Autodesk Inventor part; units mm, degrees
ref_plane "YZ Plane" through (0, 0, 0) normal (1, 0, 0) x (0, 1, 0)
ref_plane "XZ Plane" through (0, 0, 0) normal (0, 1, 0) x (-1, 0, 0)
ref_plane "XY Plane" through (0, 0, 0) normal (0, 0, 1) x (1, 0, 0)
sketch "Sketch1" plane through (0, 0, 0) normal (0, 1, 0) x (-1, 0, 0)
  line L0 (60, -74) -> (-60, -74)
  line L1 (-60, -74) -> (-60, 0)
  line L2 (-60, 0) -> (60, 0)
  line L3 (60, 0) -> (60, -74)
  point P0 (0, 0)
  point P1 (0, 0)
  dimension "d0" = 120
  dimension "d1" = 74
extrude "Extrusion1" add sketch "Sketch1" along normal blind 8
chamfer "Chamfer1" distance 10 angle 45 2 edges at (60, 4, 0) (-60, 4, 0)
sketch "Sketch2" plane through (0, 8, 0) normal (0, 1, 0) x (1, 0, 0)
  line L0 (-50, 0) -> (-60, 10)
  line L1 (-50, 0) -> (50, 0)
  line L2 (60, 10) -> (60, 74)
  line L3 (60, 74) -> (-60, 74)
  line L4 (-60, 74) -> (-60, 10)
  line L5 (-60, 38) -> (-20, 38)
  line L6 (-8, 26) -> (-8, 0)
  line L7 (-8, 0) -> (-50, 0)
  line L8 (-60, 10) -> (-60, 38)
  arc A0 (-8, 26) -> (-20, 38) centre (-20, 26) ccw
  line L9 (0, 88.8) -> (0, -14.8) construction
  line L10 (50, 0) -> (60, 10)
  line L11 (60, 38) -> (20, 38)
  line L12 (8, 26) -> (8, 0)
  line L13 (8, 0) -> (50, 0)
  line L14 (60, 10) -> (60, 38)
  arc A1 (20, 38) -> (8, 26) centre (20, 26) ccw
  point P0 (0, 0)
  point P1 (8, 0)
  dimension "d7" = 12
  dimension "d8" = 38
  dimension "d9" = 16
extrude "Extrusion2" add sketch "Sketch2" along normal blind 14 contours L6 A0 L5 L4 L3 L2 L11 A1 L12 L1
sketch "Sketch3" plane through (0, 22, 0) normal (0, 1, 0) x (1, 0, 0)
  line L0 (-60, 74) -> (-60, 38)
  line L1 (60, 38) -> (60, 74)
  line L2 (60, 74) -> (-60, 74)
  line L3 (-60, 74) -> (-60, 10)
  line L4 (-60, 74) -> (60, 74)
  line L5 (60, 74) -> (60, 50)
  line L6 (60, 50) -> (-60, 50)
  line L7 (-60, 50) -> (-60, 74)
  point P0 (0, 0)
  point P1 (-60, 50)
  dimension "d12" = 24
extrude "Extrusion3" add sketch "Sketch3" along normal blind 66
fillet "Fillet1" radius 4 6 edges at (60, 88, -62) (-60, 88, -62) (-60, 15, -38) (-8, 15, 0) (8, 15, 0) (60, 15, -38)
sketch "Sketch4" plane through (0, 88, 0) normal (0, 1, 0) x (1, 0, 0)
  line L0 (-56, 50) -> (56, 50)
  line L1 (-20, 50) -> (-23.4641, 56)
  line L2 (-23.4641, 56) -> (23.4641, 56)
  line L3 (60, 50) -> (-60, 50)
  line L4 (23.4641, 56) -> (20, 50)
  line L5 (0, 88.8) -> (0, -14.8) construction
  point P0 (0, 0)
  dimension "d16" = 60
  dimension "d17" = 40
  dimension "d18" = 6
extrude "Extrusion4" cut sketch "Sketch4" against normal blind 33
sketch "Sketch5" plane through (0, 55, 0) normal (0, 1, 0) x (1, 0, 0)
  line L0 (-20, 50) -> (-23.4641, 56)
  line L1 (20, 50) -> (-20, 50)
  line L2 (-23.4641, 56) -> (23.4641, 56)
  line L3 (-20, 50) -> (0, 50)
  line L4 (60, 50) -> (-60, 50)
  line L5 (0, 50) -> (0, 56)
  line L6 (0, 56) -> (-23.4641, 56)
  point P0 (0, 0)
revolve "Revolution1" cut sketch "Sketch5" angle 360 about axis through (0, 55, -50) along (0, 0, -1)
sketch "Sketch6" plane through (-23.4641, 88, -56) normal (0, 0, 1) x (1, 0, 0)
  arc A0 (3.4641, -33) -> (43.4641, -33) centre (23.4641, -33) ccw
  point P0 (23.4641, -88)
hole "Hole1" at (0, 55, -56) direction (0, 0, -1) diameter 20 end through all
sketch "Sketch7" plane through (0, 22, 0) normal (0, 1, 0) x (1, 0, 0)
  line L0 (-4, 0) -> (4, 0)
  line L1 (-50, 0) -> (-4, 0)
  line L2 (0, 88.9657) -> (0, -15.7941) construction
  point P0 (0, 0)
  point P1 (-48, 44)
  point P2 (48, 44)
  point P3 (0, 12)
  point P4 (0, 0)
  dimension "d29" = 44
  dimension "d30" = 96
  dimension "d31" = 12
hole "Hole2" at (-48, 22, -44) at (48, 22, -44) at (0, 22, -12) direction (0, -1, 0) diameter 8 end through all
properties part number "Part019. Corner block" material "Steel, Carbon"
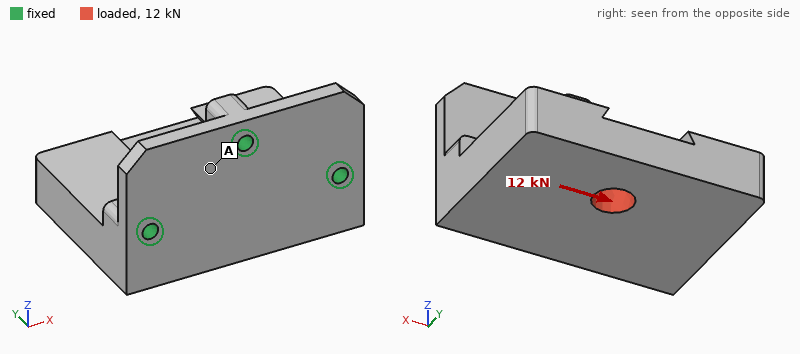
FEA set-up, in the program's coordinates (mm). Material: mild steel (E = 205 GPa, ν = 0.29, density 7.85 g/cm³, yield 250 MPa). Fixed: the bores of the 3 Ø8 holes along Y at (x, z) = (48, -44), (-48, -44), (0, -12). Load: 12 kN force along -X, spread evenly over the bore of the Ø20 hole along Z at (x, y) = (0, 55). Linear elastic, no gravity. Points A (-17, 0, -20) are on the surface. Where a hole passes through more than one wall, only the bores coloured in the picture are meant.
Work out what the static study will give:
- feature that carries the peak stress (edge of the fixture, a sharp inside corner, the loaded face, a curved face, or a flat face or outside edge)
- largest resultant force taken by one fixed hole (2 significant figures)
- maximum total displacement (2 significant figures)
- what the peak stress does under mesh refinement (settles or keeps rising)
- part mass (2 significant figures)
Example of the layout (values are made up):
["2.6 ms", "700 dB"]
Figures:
["edge of the fixture", "8.0 kN", "10 µm", "keeps rising", "2.4 kg"]
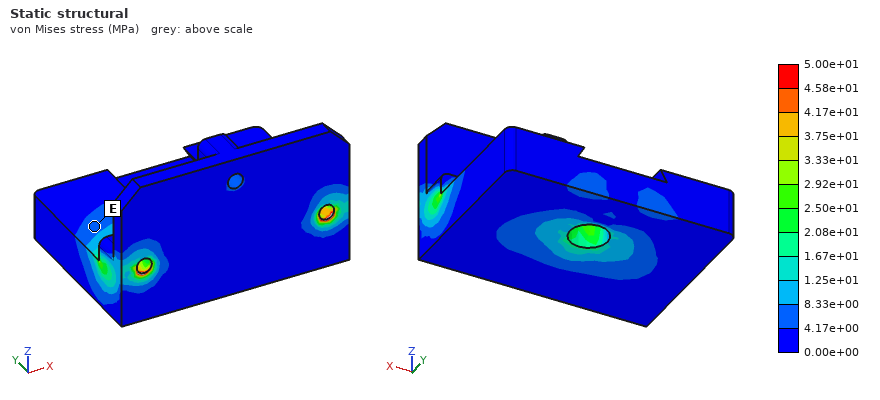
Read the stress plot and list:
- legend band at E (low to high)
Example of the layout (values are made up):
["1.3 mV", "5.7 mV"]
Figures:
["4.17e+00 to 8.33e+00 MPa"]
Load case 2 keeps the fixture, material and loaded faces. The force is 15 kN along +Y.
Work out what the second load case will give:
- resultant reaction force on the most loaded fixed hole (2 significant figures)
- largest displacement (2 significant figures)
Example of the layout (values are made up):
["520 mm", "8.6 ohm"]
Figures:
["7.9 kN", "32 µm"]
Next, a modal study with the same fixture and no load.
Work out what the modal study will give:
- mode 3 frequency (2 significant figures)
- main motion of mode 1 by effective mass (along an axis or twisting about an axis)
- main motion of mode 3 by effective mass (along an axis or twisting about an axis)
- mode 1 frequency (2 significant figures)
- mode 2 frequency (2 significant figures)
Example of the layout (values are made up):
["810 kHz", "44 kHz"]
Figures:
["6000 Hz", "along Z", "along X", "2100 Hz", "4000 Hz"]
